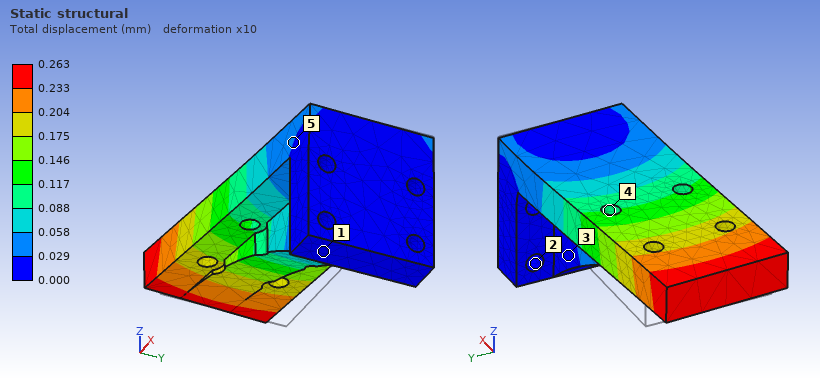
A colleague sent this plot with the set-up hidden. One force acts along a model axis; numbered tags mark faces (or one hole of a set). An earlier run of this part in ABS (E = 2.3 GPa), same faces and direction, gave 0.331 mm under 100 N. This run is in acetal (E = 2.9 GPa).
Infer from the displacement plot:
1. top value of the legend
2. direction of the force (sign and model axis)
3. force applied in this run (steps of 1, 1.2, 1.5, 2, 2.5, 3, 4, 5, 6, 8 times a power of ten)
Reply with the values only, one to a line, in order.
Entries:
0.263 mm
-Y
100 N
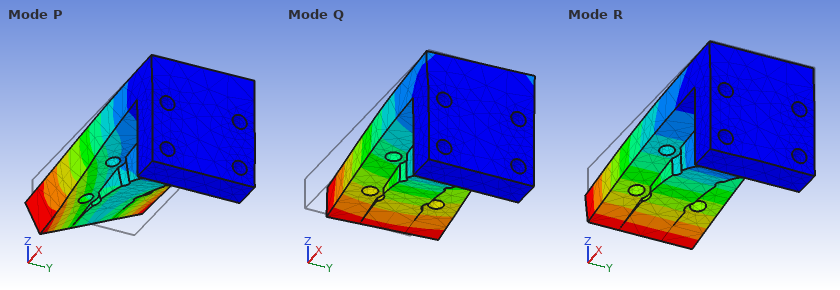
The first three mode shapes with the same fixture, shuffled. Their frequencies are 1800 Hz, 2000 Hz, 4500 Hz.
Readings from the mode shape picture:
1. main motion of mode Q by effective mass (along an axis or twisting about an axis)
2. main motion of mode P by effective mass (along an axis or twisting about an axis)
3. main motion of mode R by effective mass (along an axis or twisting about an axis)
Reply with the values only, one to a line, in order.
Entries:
along Y
twisting about X
along Z
